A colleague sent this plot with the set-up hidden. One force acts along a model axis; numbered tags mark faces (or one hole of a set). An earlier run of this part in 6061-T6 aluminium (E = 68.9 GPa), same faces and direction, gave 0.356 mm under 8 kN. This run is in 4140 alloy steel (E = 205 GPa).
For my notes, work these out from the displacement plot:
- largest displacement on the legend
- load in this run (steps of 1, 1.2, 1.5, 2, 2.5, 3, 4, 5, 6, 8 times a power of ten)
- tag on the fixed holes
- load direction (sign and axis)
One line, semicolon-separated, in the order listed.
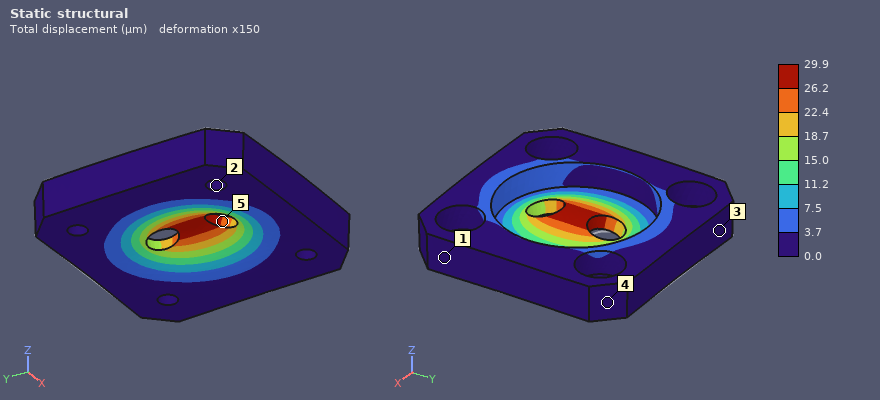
29.9 µm; 2 kN; 2; +Z
